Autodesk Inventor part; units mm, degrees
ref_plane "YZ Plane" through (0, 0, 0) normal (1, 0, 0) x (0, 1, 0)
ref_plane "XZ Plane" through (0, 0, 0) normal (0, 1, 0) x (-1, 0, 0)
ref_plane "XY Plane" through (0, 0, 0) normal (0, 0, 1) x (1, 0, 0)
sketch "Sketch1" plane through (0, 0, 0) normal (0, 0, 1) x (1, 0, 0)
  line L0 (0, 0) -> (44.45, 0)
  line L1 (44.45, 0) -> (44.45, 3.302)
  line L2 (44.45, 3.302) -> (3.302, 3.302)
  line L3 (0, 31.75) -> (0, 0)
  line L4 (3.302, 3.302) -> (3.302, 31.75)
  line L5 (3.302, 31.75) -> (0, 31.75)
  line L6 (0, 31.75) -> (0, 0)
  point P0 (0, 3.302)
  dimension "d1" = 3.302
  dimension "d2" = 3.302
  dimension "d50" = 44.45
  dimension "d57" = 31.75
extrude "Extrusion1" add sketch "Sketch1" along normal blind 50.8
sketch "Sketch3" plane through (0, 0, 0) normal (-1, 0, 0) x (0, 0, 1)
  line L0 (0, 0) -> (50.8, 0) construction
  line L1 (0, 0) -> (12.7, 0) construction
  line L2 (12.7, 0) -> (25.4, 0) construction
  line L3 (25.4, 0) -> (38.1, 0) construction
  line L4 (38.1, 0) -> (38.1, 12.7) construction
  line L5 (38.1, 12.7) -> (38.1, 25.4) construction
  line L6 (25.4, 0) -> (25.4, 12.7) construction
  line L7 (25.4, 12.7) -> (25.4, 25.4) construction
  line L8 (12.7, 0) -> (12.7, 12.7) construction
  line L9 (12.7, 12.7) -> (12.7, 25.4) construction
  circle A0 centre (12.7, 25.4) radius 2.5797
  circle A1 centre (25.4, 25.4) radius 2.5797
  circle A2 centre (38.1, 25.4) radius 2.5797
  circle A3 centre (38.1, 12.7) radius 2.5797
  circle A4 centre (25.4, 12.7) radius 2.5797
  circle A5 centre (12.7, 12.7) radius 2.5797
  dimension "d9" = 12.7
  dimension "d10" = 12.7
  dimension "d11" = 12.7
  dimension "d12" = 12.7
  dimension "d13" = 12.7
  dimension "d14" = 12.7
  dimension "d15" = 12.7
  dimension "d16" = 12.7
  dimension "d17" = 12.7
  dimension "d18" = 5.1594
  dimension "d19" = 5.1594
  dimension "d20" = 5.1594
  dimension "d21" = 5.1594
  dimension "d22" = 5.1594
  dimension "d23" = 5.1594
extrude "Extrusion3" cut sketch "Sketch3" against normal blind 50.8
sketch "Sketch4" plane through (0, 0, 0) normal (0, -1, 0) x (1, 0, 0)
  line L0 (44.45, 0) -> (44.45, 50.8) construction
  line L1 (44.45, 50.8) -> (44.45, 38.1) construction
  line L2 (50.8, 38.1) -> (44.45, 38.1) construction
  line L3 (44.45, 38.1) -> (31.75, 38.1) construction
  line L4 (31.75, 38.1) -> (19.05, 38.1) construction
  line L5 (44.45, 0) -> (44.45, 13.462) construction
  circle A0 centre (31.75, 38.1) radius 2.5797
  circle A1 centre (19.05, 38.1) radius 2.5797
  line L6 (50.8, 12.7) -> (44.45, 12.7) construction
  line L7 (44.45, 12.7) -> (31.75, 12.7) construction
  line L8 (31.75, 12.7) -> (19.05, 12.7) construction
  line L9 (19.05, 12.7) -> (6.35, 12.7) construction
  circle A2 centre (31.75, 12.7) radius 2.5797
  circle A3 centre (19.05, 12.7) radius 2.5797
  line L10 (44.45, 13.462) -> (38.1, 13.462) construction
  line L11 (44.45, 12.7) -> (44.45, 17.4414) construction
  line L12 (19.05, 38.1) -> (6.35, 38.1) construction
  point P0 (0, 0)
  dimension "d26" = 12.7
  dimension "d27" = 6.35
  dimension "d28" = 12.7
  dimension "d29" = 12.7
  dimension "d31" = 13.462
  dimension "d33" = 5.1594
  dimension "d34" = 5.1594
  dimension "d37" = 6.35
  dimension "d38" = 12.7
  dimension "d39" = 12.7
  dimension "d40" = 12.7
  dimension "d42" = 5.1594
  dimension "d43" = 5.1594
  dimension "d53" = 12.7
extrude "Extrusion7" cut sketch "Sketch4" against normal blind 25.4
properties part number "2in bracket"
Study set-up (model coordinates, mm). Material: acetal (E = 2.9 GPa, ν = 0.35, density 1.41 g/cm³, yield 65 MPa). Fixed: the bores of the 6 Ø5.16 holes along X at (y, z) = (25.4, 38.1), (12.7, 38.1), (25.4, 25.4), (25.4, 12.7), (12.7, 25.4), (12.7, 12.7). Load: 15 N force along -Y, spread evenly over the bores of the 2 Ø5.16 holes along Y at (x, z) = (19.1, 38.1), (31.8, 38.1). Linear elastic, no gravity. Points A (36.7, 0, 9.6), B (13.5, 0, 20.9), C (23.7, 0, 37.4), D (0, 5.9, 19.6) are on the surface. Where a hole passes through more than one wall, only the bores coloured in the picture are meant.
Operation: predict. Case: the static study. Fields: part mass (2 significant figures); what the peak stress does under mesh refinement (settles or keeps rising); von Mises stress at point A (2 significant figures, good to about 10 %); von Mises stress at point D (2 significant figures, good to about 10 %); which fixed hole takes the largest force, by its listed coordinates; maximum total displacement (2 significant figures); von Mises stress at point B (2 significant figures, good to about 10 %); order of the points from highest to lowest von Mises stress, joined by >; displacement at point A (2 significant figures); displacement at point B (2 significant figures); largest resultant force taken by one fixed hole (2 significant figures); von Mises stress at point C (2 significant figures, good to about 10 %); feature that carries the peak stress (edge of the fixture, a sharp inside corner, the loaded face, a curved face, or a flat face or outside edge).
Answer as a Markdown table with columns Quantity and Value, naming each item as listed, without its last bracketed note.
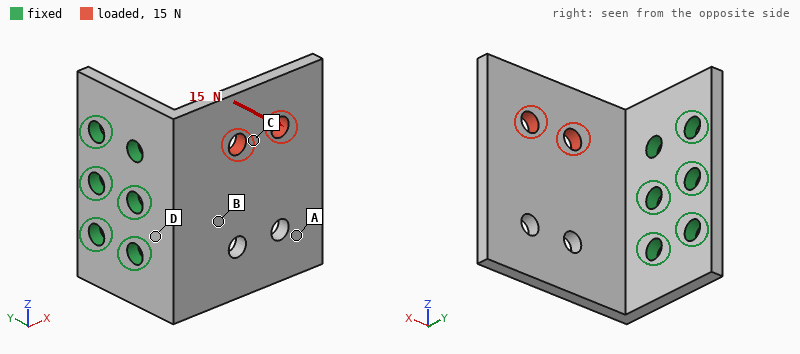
| Quantity | Value |
|---|---|
| part mass | 16 g |
| what the peak stress does under mesh refinement | keeps rising |
| von Mises stress at point A | 0.65 MPa |
| von Mises stress at point D | 3.2 MPa |
| which fixed hole takes the largest force, by its listed coordinates | (12.7, 38.1) |
| maximum total displacement | 0.75 mm |
| von Mises stress at point B | 2.2 MPa |
| order of the points from highest to lowest von Mises stress, joined by > | D > B > C > A |
| displacement at point A | 0.40 mm |
| displacement at point B | 0.13 mm |
| largest resultant force taken by one fixed hole | 10.0 N |
| von Mises stress at point C | 1.4 MPa |
| feature that carries the peak stress | edge of the fixture |
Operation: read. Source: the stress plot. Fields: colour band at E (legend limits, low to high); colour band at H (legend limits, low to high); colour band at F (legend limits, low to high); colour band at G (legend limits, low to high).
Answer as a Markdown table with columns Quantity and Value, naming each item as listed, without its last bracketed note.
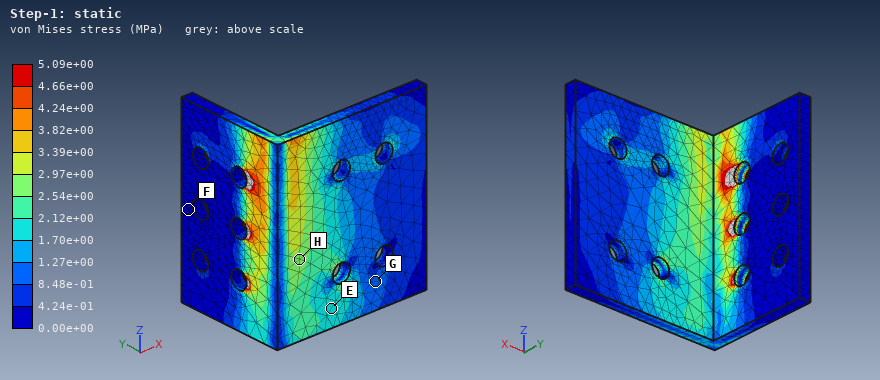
| Quantity | Value |
|---|---|
| colour band at E | 1.70e+00 to 2.12e+00 MPa |
| colour band at H | 2.54e+00 to 2.97e+00 MPa |
| colour band at F | 0.00e+00 to 4.24e-01 MPa |
| colour band at G | 8.48e-01 to 1.27e+00 MPa |
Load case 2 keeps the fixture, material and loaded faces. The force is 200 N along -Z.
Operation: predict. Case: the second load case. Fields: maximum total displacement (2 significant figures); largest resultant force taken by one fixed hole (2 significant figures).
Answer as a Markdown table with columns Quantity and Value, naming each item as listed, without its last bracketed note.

| Quantity | Value |
|---|---|
| maximum total displacement | 0.88 mm |
| largest resultant force taken by one fixed hole | 190 N |
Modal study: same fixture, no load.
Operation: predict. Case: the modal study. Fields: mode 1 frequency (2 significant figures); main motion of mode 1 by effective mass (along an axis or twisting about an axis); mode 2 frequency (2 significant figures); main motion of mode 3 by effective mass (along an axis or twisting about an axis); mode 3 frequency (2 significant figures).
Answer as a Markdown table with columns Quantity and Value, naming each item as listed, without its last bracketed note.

| Quantity | Value |
|---|---|
| mode 1 frequency | 320 Hz |
| main motion of mode 1 by effective mass | along Y |
| mode 2 frequency | 730 Hz |
| main motion of mode 3 by effective mass | along Z |
| mode 3 frequency | 1100 Hz |
